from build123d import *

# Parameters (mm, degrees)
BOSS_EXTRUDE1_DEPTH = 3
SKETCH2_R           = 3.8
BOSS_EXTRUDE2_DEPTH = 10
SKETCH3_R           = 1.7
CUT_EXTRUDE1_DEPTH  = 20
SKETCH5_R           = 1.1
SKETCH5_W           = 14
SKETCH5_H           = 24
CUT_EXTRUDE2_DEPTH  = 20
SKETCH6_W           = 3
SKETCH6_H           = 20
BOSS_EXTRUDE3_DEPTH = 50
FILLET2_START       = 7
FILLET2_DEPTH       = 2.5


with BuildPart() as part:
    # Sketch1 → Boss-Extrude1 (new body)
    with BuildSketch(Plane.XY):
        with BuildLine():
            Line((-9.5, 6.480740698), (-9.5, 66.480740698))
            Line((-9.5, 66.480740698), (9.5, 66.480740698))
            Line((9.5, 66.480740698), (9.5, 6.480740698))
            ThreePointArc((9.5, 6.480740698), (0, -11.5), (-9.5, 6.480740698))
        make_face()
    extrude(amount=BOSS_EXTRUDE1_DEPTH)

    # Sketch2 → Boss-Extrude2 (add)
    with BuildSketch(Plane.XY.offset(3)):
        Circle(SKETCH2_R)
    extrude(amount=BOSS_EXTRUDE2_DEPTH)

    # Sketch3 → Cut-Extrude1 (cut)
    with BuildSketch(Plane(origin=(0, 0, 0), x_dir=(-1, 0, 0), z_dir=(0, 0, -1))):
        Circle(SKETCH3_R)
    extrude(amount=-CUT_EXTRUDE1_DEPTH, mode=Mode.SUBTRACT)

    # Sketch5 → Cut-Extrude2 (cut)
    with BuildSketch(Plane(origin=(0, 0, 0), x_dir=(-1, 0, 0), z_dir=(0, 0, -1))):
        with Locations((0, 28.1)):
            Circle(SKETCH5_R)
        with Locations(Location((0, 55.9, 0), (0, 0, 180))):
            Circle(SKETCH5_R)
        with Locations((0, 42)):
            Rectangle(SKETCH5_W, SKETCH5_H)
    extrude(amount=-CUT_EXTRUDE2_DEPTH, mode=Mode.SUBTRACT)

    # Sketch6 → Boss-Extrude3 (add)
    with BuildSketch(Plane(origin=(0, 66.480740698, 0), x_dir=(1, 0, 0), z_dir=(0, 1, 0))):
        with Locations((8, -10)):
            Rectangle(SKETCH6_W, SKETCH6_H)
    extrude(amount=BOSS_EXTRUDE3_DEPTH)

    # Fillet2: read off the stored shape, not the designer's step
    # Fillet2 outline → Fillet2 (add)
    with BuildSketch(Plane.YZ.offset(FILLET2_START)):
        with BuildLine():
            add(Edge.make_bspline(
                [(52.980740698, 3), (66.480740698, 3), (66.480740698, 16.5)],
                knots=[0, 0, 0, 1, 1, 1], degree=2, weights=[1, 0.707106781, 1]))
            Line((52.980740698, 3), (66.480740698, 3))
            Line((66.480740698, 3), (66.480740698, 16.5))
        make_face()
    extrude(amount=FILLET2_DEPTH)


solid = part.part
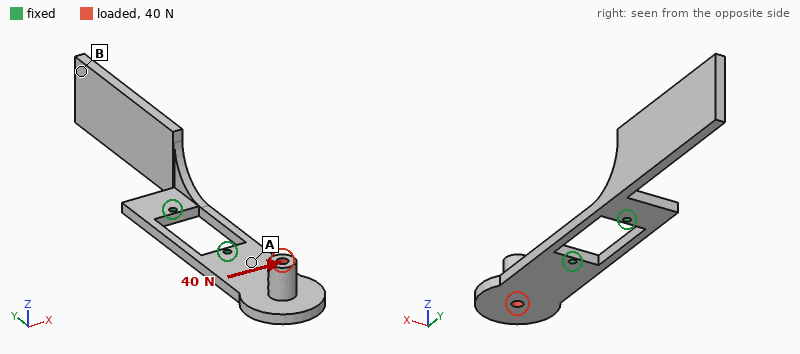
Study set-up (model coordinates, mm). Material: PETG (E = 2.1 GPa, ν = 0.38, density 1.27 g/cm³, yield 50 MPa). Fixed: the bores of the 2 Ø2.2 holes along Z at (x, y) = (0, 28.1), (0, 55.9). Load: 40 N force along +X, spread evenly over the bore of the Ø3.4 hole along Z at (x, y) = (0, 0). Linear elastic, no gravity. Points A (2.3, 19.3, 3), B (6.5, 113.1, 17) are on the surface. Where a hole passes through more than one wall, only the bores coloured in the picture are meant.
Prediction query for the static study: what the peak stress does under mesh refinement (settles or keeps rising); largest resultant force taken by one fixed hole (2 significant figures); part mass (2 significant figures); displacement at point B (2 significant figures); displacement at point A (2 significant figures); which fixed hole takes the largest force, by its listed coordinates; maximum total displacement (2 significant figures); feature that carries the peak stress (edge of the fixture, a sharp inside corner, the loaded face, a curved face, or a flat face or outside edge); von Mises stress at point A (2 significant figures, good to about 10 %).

keeps rising
45 N
8.7 g
0.75 mm
0.22 mm
(0, 28.1)
1.3 mm
edge of the fixture
8.3 MPa
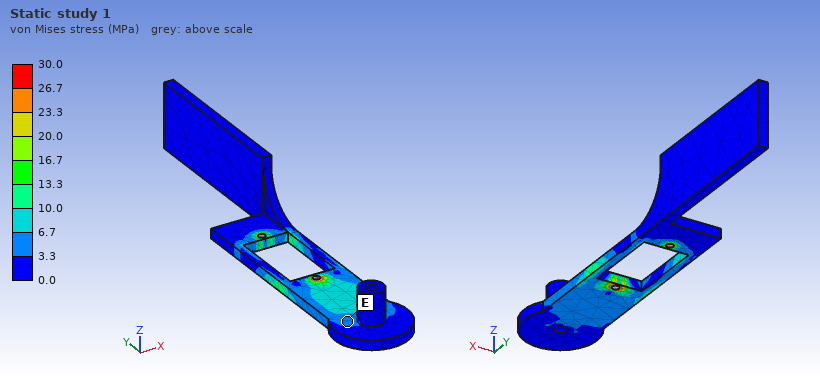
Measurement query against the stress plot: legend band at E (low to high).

3.3 to 6.7 MPa
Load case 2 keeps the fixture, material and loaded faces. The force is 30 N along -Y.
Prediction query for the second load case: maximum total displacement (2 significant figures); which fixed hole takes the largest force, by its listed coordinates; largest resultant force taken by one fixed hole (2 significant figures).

1.3 mm
(0, 28.1)
27 N
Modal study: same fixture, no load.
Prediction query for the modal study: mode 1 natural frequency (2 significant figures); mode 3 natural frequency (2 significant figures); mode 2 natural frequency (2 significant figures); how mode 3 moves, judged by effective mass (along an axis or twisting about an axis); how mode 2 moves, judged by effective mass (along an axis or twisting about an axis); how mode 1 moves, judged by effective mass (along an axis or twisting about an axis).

150 Hz
340 Hz
180 Hz
along Z
along Z
along X
